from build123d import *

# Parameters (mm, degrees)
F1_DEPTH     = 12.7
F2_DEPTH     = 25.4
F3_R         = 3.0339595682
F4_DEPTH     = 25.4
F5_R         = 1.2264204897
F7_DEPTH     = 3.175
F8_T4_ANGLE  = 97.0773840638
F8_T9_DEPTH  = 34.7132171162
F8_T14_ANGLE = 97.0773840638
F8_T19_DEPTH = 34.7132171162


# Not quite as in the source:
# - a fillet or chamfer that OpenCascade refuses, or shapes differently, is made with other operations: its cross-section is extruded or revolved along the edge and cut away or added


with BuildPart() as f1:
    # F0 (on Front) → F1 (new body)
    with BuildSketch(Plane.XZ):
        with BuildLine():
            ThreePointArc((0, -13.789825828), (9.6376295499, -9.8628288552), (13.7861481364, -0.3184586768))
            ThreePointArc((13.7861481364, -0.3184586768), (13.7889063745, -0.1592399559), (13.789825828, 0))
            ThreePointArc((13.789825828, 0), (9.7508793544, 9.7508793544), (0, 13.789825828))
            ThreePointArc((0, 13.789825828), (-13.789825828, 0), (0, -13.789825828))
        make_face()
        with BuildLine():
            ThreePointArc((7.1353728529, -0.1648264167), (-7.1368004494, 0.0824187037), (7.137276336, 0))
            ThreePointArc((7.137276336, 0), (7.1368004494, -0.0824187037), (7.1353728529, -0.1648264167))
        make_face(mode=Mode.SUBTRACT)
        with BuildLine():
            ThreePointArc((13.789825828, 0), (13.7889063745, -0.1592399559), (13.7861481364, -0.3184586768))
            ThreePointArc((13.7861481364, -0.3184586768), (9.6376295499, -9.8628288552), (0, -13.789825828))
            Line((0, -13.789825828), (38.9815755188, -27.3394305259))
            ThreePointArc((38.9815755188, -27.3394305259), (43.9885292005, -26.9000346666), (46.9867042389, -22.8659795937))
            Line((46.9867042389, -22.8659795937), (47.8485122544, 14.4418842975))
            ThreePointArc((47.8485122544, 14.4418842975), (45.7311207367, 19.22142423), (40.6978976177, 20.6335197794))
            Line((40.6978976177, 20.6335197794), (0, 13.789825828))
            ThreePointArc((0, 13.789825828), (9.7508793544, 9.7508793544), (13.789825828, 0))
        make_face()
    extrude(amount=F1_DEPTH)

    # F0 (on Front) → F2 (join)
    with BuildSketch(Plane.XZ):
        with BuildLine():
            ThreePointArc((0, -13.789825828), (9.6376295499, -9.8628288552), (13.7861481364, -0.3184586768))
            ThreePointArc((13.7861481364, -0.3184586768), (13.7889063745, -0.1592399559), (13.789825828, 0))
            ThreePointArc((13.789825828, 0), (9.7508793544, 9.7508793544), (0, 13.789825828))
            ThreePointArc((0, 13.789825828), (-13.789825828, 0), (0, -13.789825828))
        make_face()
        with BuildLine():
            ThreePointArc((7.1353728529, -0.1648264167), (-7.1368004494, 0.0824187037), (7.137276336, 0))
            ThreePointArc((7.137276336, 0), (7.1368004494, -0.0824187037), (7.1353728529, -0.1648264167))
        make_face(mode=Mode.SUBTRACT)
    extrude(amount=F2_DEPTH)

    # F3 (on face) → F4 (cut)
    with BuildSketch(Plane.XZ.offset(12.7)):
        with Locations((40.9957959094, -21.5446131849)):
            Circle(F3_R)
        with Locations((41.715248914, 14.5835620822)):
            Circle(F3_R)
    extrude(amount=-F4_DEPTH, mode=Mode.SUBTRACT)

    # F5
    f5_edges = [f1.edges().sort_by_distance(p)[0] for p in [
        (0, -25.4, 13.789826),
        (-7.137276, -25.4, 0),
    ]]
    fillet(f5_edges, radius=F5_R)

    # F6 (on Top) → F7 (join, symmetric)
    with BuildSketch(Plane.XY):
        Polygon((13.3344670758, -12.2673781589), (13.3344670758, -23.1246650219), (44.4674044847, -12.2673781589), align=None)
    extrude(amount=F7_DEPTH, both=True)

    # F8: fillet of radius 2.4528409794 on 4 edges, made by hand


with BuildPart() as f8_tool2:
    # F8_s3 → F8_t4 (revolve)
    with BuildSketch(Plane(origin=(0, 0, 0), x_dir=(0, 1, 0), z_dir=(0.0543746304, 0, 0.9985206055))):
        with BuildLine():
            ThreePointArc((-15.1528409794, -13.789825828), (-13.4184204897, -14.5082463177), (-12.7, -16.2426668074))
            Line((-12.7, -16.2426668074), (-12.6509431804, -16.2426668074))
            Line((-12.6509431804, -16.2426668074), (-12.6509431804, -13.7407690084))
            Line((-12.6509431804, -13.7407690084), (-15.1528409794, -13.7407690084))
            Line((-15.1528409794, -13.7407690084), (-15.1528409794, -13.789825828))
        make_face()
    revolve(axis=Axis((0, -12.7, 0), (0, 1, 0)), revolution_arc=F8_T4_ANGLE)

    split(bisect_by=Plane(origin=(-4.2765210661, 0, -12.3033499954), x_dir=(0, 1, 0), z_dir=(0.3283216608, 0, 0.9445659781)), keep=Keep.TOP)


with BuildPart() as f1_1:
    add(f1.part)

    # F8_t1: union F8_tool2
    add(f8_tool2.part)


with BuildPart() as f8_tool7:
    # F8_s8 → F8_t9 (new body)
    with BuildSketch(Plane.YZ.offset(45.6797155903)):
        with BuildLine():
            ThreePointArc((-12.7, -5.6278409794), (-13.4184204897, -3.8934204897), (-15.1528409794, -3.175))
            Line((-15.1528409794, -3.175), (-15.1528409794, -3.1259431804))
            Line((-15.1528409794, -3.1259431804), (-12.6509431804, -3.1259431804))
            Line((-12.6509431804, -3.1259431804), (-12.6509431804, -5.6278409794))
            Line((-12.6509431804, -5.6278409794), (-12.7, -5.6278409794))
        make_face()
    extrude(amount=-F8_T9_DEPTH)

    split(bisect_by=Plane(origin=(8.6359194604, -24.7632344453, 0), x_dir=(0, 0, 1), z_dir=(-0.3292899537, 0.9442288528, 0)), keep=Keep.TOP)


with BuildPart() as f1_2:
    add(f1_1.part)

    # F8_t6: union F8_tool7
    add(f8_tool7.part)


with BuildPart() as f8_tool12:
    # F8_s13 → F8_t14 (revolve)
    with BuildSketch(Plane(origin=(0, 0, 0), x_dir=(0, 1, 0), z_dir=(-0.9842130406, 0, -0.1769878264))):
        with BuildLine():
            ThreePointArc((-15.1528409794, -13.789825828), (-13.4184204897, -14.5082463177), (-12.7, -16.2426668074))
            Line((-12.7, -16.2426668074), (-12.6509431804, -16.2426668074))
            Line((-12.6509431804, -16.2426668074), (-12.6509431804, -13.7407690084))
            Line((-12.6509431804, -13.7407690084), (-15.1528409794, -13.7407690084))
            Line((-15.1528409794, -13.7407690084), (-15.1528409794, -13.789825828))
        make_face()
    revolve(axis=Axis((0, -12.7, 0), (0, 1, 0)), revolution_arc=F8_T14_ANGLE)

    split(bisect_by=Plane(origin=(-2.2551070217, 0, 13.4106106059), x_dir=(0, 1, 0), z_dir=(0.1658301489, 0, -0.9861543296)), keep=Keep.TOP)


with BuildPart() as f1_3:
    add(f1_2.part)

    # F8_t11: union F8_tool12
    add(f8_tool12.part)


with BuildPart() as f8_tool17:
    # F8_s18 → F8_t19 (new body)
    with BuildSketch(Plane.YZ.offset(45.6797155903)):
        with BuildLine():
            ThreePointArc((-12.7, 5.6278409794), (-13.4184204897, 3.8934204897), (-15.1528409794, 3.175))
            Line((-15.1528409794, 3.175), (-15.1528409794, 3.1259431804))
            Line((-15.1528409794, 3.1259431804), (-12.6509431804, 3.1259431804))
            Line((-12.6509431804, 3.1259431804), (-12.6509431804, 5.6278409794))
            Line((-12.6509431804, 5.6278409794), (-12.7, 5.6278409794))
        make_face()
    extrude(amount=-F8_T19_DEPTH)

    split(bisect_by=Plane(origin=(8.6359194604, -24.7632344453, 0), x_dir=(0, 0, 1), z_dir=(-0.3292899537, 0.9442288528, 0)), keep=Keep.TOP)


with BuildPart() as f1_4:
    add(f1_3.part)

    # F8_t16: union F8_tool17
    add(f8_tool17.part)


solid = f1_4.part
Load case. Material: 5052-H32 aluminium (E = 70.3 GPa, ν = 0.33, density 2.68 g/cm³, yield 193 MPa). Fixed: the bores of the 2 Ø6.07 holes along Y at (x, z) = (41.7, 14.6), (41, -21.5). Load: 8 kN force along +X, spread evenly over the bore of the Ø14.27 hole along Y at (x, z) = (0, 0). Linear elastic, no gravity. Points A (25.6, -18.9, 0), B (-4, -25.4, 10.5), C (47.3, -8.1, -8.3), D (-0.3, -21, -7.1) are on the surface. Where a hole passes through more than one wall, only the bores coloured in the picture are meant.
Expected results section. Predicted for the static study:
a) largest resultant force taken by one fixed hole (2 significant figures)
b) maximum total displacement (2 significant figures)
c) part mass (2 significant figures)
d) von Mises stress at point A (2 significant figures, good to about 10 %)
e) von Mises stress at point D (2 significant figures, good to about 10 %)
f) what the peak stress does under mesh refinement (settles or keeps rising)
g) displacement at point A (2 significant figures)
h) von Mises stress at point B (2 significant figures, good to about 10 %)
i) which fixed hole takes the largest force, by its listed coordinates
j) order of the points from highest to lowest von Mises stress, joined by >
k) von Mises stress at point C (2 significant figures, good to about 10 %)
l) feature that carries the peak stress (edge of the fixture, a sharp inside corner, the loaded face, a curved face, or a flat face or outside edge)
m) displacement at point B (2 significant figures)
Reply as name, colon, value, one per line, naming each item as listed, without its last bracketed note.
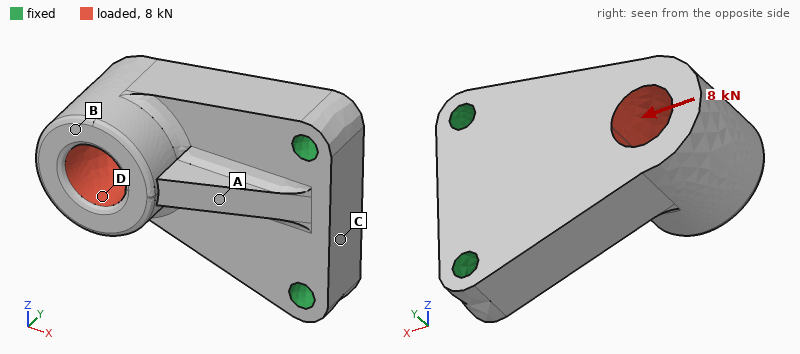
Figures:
largest resultant force taken by one fixed hole: 5.0 kN
maximum total displacement: 0.13 mm
part mass: 84 g
von Mises stress at point A: 53 MPa
von Mises stress at point D: 41 MPa
what the peak stress does under mesh refinement: keeps rising
displacement at point A: 0.034 mm
von Mises stress at point B: 11 MPa
which fixed hole takes the largest force, by its listed coordinates: (41.7, 14.6)
order of the points from highest to lowest von Mises stress, joined by >: A > D > C > B
von Mises stress at point C: 20 MPa
feature that carries the peak stress: edge of the fixture
displacement at point B: 0.10 mm
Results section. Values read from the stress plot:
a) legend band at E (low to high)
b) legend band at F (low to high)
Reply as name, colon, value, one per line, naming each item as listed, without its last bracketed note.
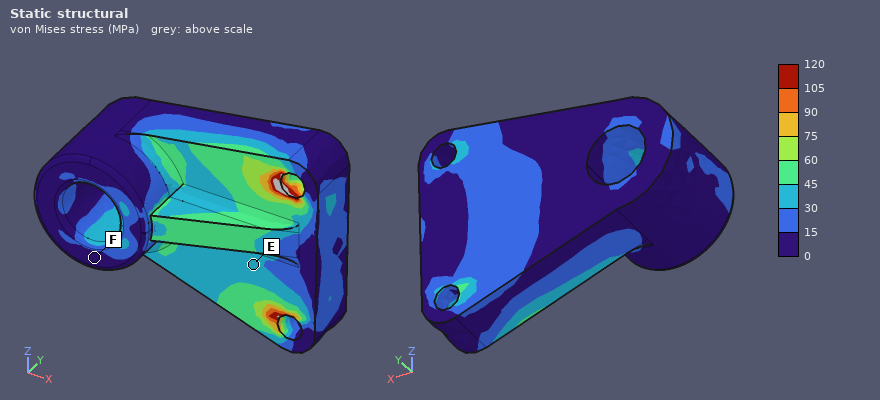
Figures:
legend band at E: 30 to 45 MPa
legend band at F: 0 to 15 MPa
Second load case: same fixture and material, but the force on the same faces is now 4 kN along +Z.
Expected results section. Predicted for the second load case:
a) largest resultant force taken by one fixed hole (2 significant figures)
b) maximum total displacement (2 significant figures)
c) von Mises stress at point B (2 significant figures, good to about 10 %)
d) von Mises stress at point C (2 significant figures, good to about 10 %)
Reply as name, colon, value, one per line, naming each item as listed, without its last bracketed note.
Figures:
largest resultant force taken by one fixed hole: 4.9 kN
maximum total displacement: 56 µm
von Mises stress at point B: 8.1 MPa
von Mises stress at point C: 4.8 MPa
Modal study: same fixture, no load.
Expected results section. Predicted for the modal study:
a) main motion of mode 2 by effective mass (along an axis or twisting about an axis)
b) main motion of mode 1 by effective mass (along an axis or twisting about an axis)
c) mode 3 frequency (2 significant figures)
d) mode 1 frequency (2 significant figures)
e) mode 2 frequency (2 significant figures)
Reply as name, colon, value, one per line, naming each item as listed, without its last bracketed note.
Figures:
main motion of mode 2 by effective mass: along Z
main motion of mode 1 by effective mass: along Y
mode 3 frequency: 12 kHz
mode 1 frequency: 3400 Hz
mode 2 frequency: 8500 Hz
